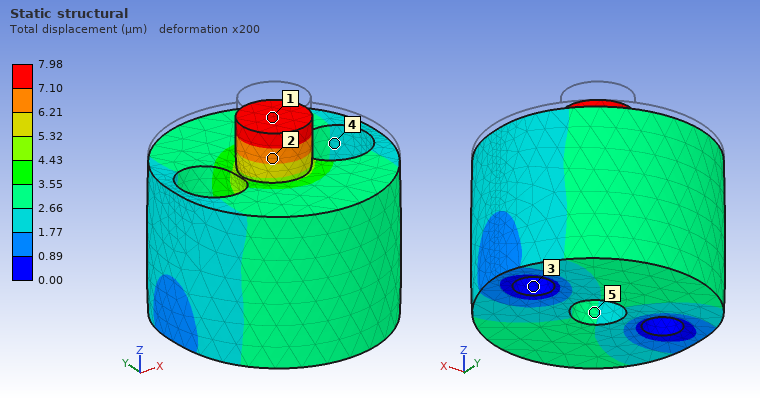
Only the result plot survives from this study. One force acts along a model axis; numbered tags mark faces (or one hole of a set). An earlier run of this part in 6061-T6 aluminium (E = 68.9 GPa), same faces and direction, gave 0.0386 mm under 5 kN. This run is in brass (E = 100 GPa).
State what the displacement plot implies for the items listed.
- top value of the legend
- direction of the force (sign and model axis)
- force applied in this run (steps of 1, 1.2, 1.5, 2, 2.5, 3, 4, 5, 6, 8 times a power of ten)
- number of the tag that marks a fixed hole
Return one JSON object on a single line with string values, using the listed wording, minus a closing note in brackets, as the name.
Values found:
{"top value of the legend": "7.98 µm", "direction of the force": "-Z", "force applied in this run": "1.5 kN", "number of the tag that marks a fixed hole": "3"}
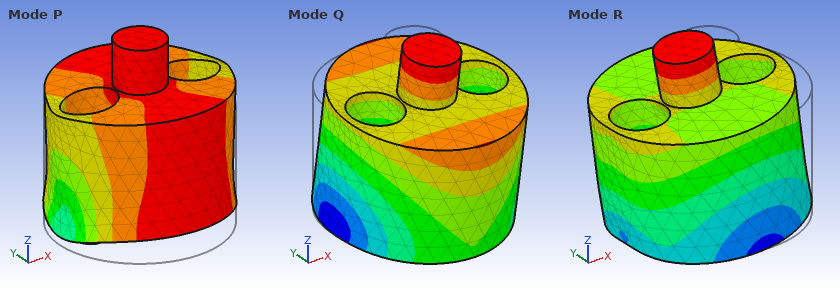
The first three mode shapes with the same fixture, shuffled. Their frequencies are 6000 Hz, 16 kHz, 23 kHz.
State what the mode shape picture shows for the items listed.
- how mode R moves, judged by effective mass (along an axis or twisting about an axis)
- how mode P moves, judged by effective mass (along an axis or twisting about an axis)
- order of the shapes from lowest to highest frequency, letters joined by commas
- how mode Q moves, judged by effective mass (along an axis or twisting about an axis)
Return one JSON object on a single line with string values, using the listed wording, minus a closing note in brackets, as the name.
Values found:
{"how mode R moves, judged by effective mass": "along X", "how mode P moves, judged by effective mass": "along Z", "order of the shapes from lowest to highest frequency, letters joined by commas": "Q, R, P", "how mode Q moves, judged by effective mass": "along Y"}
